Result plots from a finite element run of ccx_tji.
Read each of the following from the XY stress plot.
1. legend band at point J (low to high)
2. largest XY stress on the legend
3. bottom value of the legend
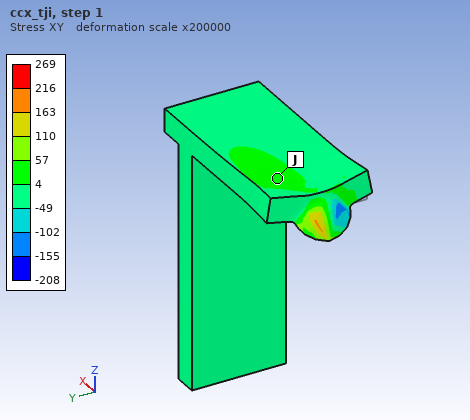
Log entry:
4 to 57
269
-208
